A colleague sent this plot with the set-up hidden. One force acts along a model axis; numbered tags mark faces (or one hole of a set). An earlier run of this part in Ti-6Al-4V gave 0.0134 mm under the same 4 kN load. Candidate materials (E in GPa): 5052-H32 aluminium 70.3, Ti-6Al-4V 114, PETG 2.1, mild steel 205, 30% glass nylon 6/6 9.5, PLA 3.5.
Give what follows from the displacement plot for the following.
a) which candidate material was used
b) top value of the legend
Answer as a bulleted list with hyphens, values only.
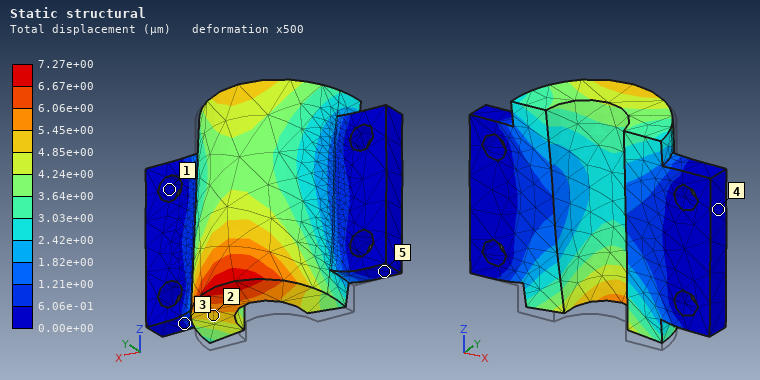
- mild steel
- 7.27e+00 µm
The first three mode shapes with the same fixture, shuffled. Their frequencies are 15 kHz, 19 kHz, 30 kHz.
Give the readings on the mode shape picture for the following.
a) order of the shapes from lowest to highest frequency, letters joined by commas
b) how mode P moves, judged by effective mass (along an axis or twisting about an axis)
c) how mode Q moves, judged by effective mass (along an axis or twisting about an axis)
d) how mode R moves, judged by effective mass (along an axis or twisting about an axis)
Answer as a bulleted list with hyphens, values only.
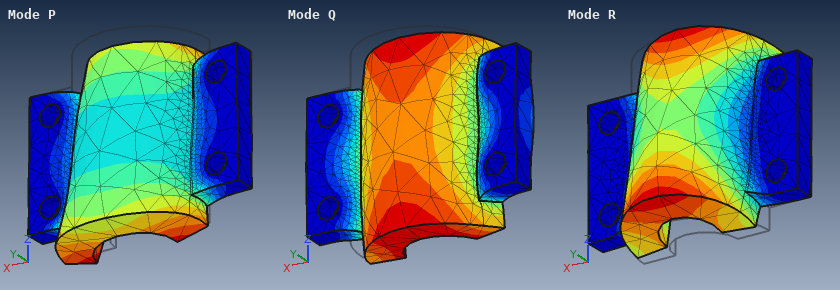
- R, Q, P
- along Z
- along Y
- along Z
